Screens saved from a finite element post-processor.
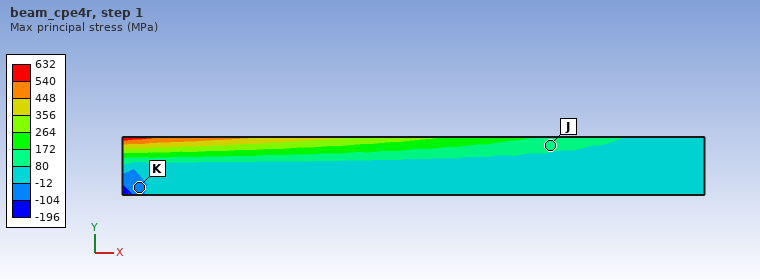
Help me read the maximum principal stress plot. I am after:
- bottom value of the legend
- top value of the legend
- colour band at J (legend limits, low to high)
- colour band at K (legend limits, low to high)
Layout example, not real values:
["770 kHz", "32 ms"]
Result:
["-196 MPa", "632 MPa", "80 to 172 MPa", "-104 to -12 MPa"]
